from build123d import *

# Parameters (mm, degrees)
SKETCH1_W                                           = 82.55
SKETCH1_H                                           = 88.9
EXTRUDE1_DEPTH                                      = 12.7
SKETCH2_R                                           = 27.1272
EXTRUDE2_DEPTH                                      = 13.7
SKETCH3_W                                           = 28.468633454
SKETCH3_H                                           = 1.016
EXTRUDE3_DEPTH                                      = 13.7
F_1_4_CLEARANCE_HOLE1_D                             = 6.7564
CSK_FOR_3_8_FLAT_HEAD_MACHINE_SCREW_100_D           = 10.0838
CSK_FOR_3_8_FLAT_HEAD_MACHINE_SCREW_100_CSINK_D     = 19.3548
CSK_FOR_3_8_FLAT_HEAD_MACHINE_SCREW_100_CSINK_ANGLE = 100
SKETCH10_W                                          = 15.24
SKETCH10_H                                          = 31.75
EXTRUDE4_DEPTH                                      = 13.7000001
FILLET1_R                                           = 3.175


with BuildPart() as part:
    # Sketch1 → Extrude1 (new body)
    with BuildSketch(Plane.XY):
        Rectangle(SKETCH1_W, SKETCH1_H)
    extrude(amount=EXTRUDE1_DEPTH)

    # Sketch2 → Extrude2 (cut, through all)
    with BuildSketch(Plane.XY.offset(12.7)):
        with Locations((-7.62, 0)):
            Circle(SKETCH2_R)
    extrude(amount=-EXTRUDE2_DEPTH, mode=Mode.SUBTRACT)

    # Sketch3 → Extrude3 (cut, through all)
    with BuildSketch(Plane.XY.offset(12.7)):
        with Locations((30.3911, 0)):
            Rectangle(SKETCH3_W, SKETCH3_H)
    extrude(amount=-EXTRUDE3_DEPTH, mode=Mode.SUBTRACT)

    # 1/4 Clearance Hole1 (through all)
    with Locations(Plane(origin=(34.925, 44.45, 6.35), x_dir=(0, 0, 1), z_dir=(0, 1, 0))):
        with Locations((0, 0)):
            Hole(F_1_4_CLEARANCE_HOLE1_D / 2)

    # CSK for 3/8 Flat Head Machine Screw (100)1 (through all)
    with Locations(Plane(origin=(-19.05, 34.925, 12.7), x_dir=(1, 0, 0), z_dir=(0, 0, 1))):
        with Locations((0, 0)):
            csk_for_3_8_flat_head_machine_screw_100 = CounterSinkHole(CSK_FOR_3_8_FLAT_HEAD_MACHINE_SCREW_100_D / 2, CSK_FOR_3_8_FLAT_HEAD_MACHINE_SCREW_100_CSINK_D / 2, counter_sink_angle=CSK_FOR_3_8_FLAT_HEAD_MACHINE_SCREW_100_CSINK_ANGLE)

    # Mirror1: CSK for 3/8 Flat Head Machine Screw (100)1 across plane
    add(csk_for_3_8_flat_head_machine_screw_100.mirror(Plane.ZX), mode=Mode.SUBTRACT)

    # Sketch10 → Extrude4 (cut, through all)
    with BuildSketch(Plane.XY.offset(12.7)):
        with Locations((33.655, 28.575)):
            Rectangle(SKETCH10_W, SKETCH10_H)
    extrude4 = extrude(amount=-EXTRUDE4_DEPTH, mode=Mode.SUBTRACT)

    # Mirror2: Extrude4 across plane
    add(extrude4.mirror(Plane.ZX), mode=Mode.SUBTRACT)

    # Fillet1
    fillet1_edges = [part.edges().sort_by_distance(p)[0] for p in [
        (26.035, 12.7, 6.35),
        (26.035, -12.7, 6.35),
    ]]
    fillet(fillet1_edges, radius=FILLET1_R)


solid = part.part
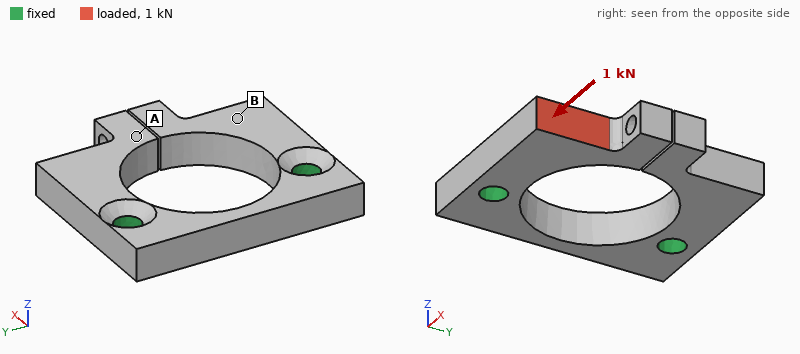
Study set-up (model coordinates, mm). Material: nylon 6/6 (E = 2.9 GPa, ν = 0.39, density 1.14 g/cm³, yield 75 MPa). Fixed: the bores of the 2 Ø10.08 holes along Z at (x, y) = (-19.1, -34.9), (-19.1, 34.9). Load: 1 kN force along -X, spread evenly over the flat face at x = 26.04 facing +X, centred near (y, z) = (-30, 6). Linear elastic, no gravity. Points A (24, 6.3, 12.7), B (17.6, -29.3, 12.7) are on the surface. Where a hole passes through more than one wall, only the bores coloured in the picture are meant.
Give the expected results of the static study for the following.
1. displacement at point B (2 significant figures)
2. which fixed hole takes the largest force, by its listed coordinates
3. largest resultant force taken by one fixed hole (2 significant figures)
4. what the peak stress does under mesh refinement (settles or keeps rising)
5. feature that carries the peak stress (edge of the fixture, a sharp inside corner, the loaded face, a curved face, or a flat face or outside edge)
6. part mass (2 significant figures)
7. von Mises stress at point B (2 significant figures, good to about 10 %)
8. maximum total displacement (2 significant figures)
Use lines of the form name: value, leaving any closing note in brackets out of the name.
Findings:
displacement at point B: 0.24 mm
which fixed hole takes the largest force, by its listed coordinates: (-19.1, -34.9)
largest resultant force taken by one fixed hole: 990 N
what the peak stress does under mesh refinement: keeps rising
feature that carries the peak stress: edge of the fixture
part mass: 54 g
von Mises stress at point B: 3.9 MPa
maximum total displacement: 0.58 mm
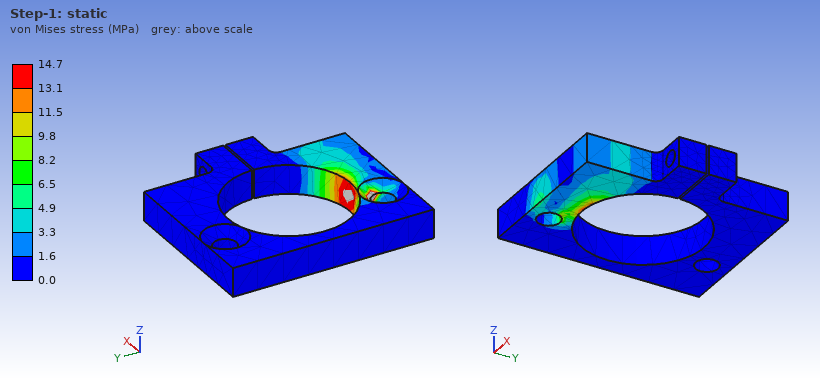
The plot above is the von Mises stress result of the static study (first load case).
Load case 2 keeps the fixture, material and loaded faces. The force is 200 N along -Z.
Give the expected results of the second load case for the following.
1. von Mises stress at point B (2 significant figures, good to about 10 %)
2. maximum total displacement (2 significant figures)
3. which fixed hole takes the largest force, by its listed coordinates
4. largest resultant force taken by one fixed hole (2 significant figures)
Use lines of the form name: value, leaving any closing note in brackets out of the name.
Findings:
von Mises stress at point B: 2.5 MPa
maximum total displacement: 1.2 mm
which fixed hole takes the largest force, by its listed coordinates: (-19.1, -34.9)
largest resultant force taken by one fixed hole: 200 N
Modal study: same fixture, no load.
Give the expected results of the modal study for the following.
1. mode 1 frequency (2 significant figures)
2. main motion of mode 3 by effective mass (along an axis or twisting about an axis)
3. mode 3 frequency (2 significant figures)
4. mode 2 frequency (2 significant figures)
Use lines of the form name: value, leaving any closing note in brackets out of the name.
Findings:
mode 1 frequency: 730 Hz
main motion of mode 3 by effective mass: along Y
mode 3 frequency: 970 Hz
mode 2 frequency: 730 Hz
